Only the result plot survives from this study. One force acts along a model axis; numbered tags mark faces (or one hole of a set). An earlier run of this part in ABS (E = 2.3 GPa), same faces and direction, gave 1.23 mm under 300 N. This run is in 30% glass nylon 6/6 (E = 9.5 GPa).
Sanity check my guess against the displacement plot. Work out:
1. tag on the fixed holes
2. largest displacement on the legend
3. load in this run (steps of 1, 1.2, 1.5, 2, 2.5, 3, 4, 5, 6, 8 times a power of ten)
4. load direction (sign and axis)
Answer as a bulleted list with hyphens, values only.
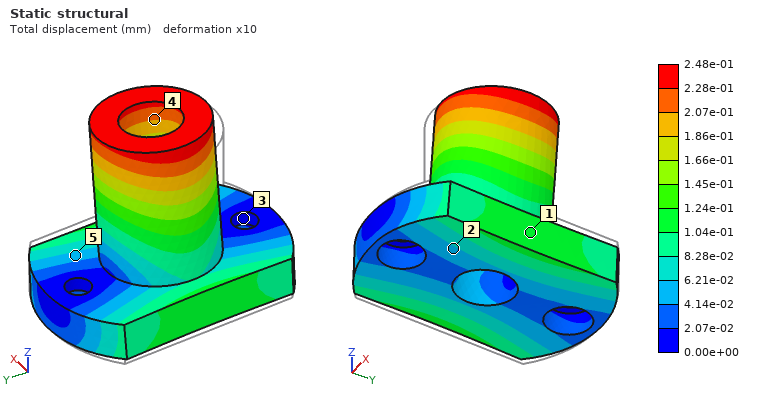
- 3
- 2.48e-01 mm
- 250 N
- +X
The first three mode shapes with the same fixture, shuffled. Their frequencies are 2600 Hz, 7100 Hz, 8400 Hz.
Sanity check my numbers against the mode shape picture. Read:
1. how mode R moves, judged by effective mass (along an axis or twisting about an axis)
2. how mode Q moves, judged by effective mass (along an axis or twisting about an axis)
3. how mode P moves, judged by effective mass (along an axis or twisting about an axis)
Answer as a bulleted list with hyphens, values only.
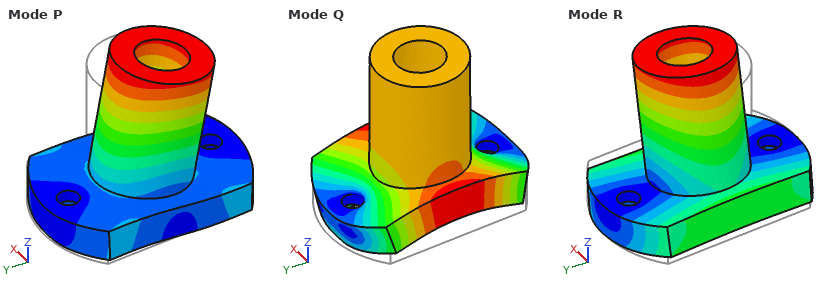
- along X
- along Z
- along Y
